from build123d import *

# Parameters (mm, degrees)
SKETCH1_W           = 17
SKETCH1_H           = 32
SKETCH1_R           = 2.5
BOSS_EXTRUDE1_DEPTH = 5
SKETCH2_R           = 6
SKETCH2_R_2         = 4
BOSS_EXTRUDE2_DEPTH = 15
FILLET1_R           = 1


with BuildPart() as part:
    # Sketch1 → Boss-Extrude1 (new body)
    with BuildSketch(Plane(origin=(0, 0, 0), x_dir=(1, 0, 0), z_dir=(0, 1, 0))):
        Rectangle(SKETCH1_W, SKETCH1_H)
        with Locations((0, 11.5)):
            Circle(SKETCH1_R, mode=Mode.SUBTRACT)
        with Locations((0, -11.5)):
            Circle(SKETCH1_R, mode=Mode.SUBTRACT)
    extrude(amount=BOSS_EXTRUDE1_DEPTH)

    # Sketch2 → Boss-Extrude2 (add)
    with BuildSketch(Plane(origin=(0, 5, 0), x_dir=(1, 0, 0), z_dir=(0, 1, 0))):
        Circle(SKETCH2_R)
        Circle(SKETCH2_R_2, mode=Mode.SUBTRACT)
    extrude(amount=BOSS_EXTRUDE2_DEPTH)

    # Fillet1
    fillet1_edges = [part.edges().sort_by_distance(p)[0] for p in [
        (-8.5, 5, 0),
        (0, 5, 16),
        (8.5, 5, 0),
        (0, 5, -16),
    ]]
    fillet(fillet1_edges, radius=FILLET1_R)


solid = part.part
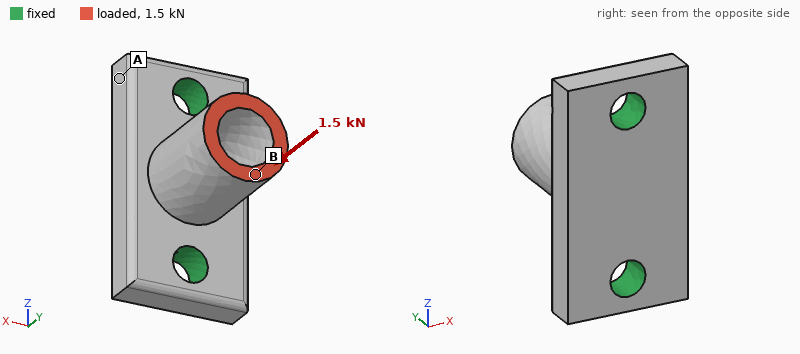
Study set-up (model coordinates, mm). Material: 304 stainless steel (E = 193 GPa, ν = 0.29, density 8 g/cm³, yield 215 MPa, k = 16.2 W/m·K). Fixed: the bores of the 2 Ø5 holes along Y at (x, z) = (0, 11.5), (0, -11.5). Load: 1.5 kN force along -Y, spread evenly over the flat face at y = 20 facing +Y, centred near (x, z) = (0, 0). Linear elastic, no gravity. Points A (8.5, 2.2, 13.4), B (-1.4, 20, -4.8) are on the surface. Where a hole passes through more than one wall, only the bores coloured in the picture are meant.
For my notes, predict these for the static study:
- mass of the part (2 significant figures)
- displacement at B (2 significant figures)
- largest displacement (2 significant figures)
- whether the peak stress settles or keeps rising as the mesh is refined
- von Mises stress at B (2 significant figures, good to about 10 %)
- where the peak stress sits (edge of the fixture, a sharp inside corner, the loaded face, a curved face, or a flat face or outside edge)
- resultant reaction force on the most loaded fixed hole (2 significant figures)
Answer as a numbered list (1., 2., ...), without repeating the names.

1. 28 g
2. 3.9 µm
3. 3.9 µm
4. keeps rising
5. 24 MPa
6. edge of the fixture
7. 760 N
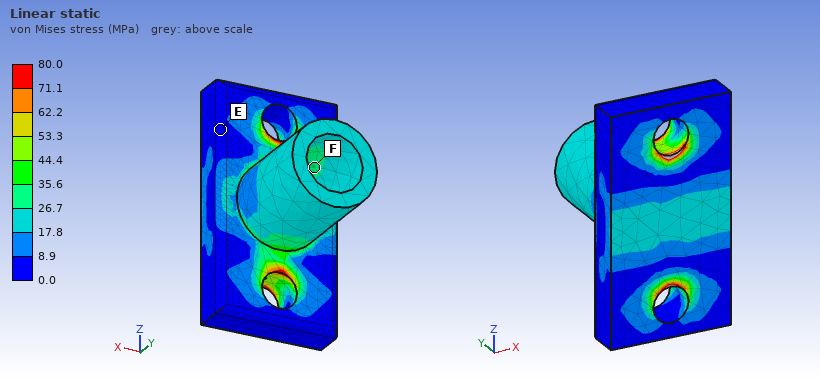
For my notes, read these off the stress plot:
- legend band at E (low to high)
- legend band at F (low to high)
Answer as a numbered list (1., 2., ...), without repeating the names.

1. 0.0 to 8.9 MPa
2. 26.7 to 35.6 MPa
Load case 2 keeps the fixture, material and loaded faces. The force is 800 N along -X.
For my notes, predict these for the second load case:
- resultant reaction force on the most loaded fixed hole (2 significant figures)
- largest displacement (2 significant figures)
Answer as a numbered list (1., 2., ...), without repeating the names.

1. 400 N
2. 31 µm
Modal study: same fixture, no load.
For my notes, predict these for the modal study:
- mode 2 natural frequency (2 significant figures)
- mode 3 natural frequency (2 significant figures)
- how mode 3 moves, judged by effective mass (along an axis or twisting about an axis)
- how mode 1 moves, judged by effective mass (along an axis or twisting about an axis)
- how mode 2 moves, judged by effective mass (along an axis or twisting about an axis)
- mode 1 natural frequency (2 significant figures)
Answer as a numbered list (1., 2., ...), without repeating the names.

1. 22 kHz
2. 32 kHz
3. along Y
4. along X
5. along Z
6. 15 kHz
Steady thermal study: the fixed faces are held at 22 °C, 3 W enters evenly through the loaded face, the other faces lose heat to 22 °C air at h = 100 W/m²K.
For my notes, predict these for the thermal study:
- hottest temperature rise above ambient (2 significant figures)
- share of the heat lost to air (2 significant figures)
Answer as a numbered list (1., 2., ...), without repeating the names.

1. 34 K
2. 60 %
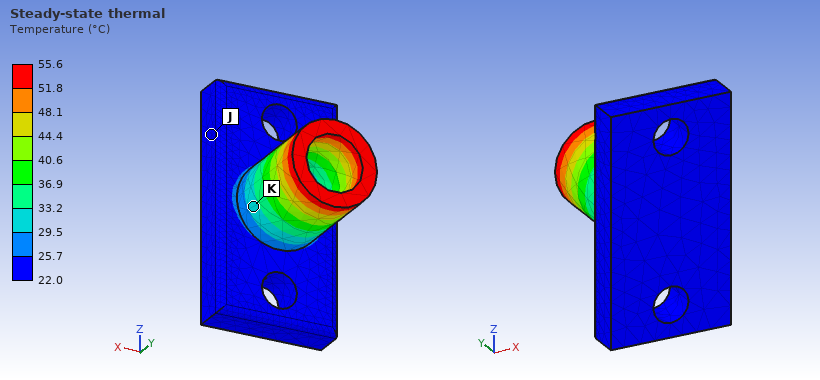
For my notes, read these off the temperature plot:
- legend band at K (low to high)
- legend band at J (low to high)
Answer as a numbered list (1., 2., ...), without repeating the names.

1. 29.5 to 33.2 °C
2. 22.0 to 25.7 °C
